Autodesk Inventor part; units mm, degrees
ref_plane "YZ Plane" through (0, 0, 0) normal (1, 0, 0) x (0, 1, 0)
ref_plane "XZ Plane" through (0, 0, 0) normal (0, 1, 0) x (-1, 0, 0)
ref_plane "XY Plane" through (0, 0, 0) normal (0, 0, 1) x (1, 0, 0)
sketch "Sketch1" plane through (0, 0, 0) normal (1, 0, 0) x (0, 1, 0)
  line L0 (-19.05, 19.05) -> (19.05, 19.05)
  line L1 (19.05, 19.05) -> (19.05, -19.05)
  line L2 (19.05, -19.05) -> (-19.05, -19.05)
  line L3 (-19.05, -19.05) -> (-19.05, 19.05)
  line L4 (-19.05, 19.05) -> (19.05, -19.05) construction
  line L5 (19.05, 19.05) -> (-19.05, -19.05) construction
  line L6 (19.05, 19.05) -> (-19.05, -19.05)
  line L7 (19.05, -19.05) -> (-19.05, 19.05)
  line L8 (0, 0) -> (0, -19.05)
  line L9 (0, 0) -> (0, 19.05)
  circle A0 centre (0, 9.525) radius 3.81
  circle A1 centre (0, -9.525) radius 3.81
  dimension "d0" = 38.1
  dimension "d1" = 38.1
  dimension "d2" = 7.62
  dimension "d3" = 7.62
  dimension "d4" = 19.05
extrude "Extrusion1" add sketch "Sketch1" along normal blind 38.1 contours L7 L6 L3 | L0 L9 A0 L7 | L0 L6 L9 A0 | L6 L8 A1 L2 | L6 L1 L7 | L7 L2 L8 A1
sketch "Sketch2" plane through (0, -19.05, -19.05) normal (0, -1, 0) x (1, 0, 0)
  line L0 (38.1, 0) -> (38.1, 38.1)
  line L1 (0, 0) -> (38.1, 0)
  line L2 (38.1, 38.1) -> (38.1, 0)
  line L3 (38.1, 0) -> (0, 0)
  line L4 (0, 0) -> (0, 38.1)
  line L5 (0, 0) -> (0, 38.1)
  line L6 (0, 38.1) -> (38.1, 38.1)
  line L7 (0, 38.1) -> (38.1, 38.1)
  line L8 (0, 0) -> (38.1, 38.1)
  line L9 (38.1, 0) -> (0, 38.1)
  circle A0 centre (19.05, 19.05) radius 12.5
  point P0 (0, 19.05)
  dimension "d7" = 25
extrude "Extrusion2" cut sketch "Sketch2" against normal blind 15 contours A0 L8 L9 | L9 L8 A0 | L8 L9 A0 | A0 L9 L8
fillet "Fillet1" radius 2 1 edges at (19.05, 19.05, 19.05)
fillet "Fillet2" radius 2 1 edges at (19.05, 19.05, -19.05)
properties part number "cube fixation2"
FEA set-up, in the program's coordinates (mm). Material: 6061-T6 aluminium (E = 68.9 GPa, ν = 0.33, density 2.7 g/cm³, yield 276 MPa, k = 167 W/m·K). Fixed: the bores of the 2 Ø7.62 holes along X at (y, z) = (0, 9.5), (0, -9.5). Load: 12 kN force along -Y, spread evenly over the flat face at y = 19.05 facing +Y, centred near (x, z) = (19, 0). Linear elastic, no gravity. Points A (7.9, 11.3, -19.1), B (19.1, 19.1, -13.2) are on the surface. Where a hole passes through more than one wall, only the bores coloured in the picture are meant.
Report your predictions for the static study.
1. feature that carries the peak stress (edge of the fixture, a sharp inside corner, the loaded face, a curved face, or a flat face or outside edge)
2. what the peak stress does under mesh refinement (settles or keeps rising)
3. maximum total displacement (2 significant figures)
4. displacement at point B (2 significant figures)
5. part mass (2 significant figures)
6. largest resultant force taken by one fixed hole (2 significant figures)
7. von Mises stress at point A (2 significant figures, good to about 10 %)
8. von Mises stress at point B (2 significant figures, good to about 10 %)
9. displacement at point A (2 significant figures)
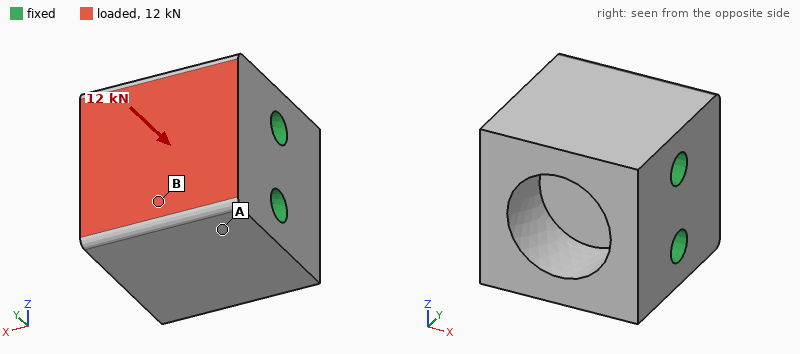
edge of the fixture
keeps rising
2.6 µm
2.1 µm
120 g
6.1 kN
3.6 MPa
7.4 MPa
1.5 µm
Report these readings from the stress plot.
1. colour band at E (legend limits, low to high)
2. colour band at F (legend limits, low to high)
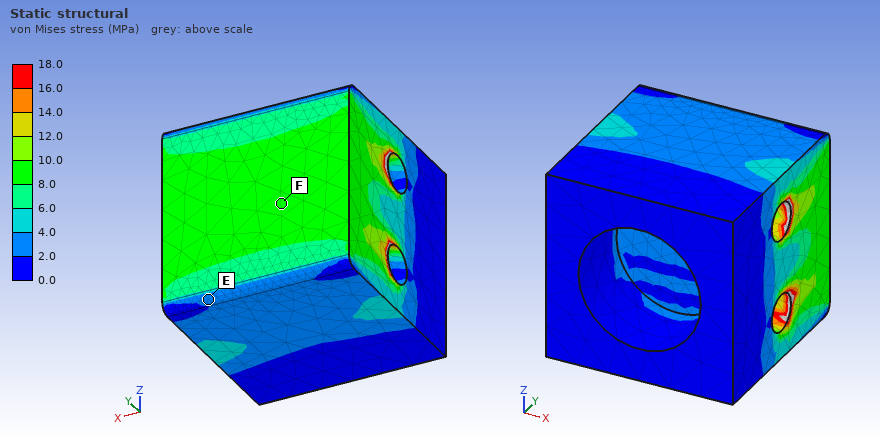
2.0 to 4.0 MPa
8.0 to 10.0 MPa
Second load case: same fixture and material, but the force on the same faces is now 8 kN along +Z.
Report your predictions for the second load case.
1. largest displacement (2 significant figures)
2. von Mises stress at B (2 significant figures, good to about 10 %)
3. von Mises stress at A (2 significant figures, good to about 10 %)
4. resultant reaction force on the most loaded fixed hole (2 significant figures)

7.2 µm
12 MPa
7.5 MPa
6.8 kN
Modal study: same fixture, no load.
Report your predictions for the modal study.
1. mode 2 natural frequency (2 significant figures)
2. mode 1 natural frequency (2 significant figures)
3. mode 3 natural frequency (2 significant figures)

32 kHz
29 kHz
33 kHz
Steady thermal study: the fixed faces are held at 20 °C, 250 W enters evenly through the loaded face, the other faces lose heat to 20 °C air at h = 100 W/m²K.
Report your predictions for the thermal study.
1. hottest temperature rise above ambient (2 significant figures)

19 K
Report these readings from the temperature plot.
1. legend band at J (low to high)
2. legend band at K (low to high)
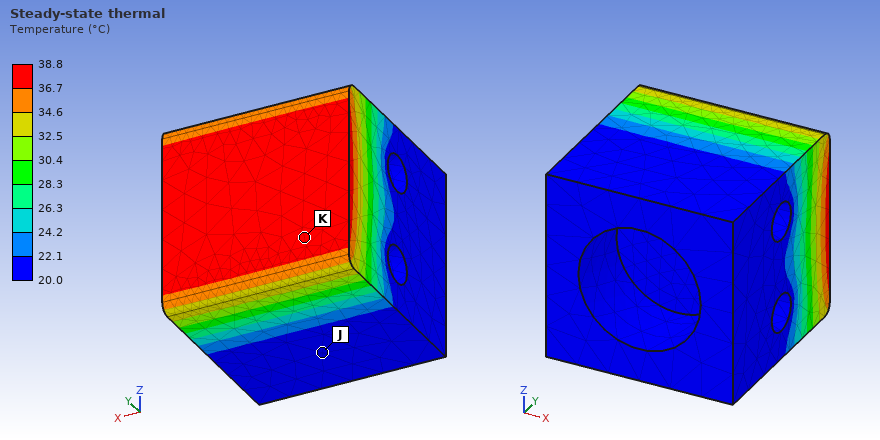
20.0 to 22.1 °C
36.7 to 38.8 °C
